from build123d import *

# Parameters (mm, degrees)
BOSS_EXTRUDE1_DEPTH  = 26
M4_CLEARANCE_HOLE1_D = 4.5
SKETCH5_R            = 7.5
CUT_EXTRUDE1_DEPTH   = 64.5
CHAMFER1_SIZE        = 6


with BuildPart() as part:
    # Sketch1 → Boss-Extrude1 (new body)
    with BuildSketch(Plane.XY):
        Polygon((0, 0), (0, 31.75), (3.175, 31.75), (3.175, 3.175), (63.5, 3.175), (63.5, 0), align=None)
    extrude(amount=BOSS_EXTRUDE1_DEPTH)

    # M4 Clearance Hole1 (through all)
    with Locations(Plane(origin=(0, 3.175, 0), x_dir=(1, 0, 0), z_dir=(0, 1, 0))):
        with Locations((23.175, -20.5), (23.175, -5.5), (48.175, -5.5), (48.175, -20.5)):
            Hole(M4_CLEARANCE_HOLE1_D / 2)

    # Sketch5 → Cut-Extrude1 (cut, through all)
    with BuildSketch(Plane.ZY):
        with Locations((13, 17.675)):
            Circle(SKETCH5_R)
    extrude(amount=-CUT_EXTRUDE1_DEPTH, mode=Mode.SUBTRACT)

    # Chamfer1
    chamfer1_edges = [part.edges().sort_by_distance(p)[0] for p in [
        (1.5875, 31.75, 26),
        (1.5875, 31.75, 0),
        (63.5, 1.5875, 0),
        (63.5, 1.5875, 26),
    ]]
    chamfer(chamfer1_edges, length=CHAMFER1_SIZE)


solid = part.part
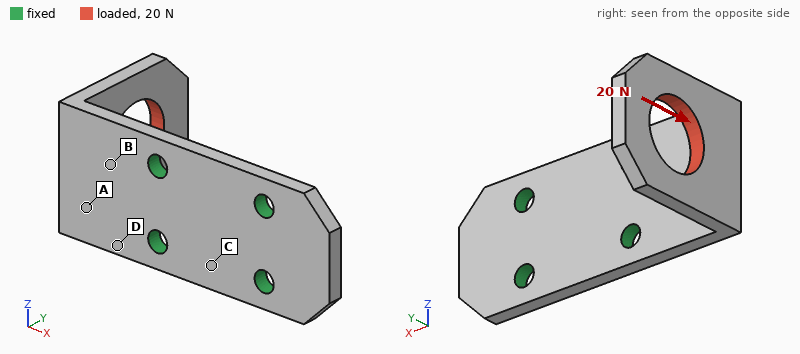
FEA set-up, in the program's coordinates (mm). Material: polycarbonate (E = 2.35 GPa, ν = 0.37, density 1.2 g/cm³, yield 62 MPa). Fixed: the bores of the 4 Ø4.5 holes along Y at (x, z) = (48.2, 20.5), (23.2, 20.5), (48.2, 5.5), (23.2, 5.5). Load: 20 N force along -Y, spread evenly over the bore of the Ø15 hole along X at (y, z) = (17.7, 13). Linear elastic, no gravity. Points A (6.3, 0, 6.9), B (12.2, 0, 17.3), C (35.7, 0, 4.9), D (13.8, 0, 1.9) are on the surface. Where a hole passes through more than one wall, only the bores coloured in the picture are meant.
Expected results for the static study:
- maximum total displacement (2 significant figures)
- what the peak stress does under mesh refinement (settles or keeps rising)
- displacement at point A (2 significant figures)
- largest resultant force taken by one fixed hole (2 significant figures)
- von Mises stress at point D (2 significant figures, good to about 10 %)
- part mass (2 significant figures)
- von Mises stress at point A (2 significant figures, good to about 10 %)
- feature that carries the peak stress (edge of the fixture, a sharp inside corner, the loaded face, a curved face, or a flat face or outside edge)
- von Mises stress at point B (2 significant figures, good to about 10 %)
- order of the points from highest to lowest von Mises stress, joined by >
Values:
0.82 mm
keeps rising
0.22 mm
10 N
5.6 MPa
7.9 g
2.1 MPa
edge of the fixture
4.3 MPa
D > B > A > C
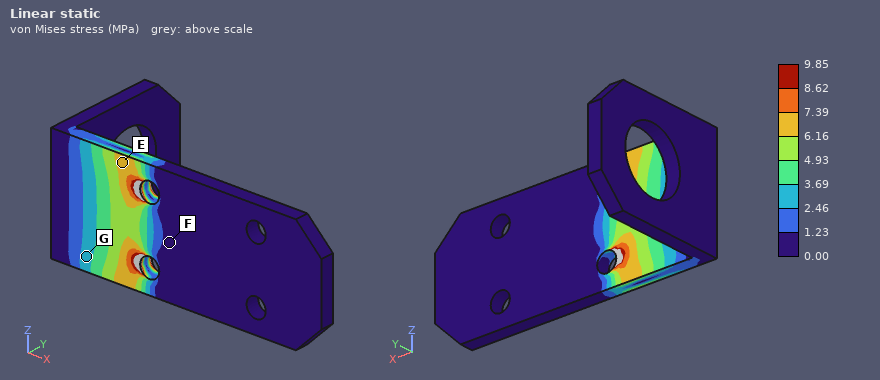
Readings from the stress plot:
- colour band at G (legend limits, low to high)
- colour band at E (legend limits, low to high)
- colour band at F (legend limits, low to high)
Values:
2.46 to 3.69 MPa
6.16 to 7.39 MPa
0.00 to 1.23 MPa
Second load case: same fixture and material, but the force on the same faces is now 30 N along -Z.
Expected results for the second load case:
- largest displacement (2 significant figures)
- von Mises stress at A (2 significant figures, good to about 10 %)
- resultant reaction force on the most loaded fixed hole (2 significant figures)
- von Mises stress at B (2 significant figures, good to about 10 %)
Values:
0.82 mm
5.8 MPa
45 N
6.1 MPa
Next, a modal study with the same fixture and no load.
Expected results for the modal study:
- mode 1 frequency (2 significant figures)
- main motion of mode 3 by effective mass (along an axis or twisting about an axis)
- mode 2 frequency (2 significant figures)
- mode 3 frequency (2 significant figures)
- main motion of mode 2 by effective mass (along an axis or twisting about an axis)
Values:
440 Hz
along Y
770 Hz
1200 Hz
along Z
